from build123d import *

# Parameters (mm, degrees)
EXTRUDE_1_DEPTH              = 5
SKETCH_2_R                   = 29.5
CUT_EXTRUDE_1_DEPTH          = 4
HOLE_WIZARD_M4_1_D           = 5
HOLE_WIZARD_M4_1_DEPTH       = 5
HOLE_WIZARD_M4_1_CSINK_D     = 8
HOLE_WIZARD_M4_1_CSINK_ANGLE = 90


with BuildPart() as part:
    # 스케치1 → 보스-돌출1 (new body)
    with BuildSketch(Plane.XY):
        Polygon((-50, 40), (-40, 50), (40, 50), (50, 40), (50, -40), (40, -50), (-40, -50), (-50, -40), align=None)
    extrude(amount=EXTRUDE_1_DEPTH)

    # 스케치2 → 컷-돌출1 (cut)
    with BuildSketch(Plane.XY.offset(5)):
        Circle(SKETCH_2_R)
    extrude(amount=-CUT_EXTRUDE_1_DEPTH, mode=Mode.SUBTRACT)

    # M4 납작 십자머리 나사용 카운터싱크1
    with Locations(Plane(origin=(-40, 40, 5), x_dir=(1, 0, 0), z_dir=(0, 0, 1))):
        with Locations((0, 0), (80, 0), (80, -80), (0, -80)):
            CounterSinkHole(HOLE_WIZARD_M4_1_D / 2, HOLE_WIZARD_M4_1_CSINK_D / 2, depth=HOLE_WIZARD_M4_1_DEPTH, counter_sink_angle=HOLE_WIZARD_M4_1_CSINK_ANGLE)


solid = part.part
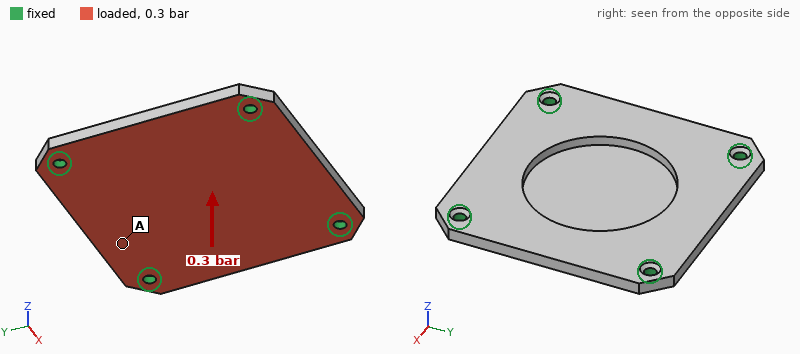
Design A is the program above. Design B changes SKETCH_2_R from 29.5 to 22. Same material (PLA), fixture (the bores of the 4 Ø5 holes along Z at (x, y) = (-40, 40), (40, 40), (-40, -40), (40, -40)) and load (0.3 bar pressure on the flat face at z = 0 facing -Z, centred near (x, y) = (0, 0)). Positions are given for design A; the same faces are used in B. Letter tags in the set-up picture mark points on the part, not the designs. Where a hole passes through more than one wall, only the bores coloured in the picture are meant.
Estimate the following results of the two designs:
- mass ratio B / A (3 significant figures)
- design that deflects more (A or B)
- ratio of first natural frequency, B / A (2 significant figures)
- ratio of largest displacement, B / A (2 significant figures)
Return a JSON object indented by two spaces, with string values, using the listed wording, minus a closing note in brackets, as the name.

{
  "mass ratio B / A": "1.13",
  "design that deflects more": "A",
  "ratio of first natural frequency, B / A": "1.1",
  "ratio of largest displacement, B / A": "0.47"
}
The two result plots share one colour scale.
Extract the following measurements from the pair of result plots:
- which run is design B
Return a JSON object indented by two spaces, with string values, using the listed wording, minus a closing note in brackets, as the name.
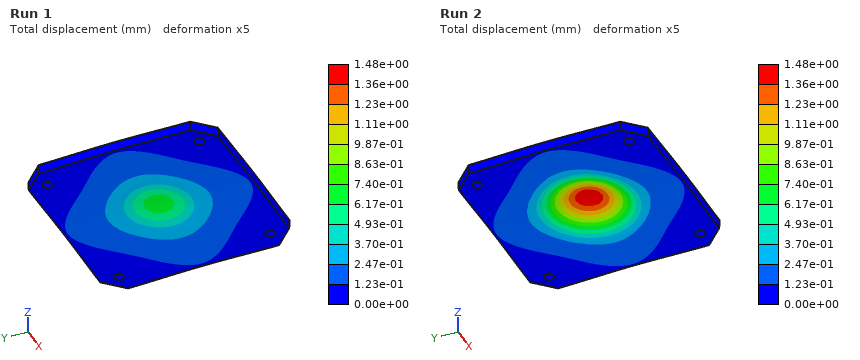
{
  "which run is design B": "Run 1"
}
